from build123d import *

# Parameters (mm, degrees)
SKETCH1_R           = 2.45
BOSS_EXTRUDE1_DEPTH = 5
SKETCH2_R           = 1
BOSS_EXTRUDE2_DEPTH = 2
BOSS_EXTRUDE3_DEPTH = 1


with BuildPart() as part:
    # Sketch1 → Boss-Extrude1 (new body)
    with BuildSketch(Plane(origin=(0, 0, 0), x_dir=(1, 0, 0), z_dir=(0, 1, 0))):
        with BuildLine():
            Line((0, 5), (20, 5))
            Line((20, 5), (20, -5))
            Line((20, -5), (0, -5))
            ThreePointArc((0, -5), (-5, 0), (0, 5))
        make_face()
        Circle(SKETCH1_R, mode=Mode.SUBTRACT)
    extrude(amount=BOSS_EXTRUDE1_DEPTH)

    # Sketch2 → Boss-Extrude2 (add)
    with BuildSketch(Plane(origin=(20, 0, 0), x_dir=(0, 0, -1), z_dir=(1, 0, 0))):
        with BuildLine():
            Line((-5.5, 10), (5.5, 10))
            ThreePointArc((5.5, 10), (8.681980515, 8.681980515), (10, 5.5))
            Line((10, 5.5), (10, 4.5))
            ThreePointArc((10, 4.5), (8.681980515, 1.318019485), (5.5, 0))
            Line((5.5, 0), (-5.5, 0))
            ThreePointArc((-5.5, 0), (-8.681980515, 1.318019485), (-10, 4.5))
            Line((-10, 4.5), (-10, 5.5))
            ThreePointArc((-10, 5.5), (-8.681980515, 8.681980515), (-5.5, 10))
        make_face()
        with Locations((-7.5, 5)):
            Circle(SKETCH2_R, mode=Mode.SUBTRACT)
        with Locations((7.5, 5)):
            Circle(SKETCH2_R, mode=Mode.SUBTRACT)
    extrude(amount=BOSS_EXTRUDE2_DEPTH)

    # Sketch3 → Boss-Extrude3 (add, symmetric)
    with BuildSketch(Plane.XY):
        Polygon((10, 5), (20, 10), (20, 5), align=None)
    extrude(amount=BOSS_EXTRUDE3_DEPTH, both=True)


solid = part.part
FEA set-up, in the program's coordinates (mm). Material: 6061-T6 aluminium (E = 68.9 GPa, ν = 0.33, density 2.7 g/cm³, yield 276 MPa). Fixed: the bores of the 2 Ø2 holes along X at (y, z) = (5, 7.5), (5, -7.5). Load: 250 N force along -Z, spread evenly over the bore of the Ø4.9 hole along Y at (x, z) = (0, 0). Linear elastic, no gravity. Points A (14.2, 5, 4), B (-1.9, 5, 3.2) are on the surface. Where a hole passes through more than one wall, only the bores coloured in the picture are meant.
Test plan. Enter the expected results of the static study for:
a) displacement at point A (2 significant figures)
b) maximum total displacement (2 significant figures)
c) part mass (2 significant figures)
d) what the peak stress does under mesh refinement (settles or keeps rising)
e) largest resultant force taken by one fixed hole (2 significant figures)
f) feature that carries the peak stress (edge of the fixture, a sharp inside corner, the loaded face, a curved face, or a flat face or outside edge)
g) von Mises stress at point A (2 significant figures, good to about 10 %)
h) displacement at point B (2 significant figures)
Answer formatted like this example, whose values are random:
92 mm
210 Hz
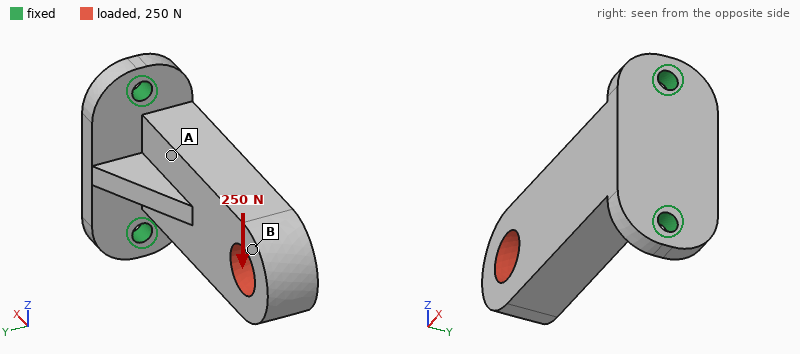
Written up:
21 µm
91 µm
4.1 g
keeps rising
450 N
edge of the fixture
40 MPa
80 µm
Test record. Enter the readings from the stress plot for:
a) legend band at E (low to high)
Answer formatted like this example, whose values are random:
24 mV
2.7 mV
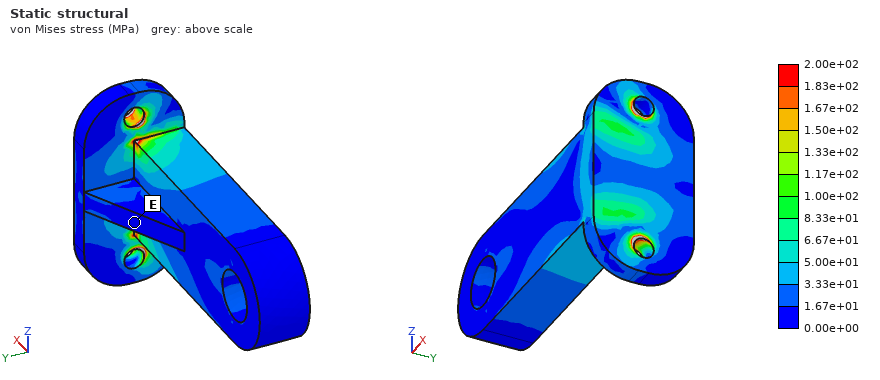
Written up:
0.00e+00 to 1.67e+01 MPa
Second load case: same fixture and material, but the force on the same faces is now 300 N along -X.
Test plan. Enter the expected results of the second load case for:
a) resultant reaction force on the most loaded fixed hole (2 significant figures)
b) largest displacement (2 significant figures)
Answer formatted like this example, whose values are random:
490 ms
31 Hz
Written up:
160 N
47 µm
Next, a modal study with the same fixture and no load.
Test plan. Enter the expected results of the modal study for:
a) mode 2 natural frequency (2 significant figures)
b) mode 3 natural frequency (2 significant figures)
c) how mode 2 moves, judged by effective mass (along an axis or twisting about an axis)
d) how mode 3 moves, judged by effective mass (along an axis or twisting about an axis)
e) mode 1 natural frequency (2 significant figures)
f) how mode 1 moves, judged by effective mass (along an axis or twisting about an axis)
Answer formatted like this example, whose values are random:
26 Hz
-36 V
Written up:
8400 Hz
21 kHz
along Z
along X
3500 Hz
along Y
